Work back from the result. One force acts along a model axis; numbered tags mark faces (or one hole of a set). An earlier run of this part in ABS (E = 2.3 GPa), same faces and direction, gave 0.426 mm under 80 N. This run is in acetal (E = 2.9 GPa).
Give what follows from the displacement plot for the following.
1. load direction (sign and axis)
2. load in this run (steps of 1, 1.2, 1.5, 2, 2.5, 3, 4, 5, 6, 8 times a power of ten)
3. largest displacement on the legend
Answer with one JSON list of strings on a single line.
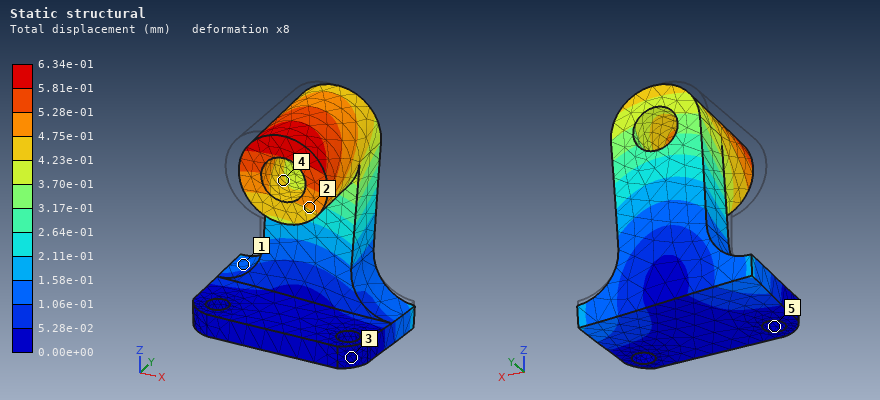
["+X", "150 N", "6.34e-01 mm"]
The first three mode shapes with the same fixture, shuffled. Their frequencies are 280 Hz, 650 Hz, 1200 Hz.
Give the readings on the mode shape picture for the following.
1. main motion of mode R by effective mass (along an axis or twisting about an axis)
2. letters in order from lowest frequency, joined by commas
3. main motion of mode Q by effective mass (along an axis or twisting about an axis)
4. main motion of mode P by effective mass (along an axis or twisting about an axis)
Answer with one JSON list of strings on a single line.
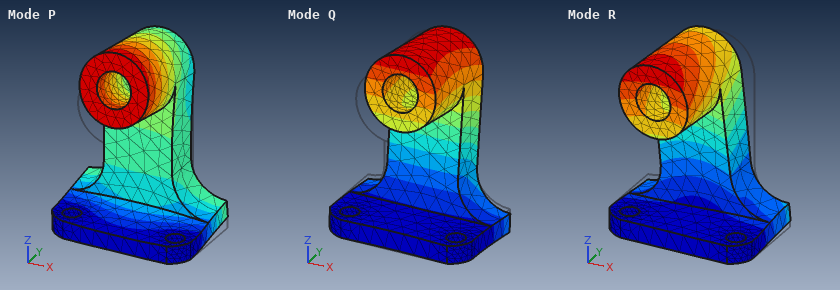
["along X", "Q, R, P", "along Y", "along Z"]
